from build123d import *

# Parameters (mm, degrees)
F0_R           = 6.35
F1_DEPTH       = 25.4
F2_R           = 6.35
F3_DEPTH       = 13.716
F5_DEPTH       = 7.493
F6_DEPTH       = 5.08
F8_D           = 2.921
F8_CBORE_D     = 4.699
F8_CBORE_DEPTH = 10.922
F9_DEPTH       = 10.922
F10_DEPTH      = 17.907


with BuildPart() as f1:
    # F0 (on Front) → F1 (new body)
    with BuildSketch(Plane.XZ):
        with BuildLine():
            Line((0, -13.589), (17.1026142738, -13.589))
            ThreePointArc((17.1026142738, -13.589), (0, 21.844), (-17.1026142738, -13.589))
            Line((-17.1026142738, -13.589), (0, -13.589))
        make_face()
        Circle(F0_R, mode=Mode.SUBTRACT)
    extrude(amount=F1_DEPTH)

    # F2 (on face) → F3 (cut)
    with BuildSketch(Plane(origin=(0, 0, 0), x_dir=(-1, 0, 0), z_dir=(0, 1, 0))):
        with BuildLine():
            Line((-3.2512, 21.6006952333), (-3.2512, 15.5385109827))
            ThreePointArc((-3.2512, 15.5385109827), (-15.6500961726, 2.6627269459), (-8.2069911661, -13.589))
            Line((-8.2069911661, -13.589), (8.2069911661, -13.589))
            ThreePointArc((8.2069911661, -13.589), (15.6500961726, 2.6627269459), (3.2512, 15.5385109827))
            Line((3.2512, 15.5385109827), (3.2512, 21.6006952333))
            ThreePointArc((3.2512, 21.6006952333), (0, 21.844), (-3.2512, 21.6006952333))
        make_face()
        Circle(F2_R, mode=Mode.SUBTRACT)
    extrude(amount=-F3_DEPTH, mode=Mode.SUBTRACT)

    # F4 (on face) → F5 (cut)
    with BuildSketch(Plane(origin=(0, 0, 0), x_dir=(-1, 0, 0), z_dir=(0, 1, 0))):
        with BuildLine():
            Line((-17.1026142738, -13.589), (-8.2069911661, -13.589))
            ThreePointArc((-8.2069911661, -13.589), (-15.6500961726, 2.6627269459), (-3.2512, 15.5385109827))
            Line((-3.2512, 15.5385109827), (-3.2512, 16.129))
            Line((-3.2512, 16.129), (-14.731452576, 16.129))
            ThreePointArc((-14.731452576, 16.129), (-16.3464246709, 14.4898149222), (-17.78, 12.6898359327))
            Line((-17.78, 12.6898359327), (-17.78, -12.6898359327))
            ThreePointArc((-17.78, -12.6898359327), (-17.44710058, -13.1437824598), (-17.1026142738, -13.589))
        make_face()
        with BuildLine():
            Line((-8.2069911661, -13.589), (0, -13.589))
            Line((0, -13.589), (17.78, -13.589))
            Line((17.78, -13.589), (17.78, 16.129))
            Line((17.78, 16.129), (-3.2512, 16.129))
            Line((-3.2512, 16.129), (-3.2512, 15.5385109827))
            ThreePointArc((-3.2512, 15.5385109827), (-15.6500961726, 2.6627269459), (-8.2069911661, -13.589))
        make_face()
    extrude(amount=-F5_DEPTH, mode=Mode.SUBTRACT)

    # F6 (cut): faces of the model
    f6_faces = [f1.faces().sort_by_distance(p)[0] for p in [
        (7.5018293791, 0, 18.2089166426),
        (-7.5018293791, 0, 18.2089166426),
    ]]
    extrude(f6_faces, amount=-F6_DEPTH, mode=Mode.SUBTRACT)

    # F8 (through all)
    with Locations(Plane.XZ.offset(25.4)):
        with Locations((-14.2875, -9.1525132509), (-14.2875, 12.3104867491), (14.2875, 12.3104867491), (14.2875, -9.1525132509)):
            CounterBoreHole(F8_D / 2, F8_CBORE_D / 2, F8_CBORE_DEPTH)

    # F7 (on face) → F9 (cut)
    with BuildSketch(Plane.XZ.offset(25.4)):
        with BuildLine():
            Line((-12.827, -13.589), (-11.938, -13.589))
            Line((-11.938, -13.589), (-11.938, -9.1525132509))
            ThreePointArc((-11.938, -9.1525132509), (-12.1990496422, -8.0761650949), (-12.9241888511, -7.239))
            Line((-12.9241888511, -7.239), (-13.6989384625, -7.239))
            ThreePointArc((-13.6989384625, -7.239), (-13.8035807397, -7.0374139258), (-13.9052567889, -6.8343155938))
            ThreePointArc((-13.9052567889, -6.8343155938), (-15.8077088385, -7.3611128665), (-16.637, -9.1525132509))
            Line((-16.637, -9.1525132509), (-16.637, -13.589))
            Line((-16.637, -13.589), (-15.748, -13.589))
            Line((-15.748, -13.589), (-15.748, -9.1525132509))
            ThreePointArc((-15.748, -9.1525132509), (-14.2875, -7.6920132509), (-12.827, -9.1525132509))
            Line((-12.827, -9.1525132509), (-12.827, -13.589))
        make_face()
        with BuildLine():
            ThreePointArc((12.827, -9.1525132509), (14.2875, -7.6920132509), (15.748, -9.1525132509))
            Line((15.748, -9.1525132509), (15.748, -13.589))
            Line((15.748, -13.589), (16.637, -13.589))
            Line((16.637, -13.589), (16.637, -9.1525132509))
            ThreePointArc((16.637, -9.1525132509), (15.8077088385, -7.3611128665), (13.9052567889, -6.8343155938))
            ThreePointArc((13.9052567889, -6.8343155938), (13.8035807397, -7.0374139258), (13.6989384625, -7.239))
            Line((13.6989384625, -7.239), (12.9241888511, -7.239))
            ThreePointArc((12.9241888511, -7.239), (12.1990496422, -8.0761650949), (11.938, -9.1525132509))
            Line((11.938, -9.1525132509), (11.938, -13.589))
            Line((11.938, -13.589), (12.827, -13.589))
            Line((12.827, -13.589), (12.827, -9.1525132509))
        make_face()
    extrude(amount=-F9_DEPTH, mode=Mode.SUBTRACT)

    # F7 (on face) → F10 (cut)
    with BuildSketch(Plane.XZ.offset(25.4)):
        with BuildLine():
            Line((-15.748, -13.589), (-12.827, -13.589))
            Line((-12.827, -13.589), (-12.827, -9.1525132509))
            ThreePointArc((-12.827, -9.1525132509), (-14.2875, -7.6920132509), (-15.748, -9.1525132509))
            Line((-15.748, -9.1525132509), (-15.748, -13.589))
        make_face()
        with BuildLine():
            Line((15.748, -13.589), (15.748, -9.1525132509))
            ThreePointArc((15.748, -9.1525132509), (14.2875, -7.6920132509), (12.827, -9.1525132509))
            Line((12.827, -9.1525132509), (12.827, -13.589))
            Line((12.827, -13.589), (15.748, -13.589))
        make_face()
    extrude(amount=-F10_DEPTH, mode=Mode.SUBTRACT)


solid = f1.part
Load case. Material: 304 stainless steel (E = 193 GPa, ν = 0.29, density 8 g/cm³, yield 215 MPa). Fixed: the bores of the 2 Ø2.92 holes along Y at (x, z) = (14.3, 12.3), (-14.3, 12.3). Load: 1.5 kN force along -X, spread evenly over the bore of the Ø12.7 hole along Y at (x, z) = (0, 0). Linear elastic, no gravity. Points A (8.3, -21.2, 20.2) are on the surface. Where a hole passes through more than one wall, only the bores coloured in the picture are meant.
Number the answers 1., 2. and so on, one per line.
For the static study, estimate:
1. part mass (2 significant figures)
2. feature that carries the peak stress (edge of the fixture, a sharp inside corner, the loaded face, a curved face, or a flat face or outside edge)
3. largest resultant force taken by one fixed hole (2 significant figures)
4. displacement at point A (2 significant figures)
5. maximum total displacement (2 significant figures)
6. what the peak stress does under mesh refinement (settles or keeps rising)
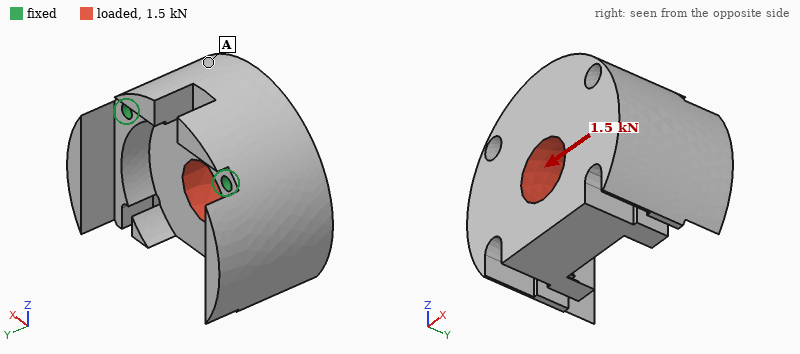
1. 130 g
2. edge of the fixture
3. 1.0 kN
4. 0.73 µm
5. 4.8 µm
6. keeps rising
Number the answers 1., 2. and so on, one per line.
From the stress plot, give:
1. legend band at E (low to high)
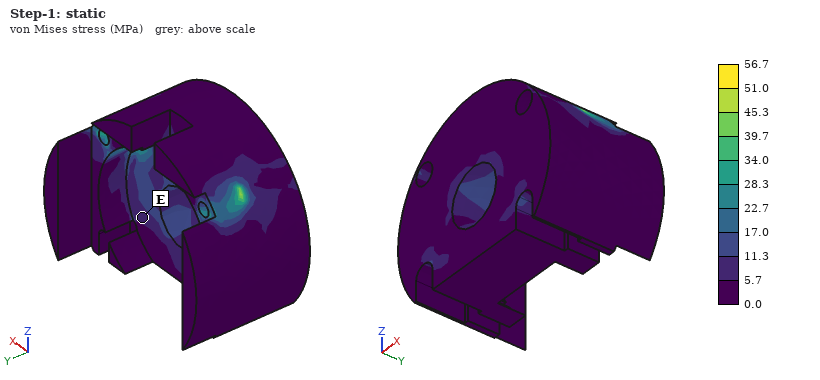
1. 5.7 to 11.3 MPa
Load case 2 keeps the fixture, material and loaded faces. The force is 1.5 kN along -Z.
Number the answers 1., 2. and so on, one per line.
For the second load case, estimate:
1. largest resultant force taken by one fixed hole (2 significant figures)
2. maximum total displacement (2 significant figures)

1. 750 N
2. 12 µm
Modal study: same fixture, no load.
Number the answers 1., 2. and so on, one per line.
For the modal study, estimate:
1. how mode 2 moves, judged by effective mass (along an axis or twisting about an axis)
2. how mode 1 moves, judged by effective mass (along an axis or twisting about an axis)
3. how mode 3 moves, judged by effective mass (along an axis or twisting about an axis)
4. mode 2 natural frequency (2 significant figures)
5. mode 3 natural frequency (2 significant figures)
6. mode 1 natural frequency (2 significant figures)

1. along X
2. along Y
3. along X
4. 9300 Hz
5. 14 kHz
6. 4800 Hz
